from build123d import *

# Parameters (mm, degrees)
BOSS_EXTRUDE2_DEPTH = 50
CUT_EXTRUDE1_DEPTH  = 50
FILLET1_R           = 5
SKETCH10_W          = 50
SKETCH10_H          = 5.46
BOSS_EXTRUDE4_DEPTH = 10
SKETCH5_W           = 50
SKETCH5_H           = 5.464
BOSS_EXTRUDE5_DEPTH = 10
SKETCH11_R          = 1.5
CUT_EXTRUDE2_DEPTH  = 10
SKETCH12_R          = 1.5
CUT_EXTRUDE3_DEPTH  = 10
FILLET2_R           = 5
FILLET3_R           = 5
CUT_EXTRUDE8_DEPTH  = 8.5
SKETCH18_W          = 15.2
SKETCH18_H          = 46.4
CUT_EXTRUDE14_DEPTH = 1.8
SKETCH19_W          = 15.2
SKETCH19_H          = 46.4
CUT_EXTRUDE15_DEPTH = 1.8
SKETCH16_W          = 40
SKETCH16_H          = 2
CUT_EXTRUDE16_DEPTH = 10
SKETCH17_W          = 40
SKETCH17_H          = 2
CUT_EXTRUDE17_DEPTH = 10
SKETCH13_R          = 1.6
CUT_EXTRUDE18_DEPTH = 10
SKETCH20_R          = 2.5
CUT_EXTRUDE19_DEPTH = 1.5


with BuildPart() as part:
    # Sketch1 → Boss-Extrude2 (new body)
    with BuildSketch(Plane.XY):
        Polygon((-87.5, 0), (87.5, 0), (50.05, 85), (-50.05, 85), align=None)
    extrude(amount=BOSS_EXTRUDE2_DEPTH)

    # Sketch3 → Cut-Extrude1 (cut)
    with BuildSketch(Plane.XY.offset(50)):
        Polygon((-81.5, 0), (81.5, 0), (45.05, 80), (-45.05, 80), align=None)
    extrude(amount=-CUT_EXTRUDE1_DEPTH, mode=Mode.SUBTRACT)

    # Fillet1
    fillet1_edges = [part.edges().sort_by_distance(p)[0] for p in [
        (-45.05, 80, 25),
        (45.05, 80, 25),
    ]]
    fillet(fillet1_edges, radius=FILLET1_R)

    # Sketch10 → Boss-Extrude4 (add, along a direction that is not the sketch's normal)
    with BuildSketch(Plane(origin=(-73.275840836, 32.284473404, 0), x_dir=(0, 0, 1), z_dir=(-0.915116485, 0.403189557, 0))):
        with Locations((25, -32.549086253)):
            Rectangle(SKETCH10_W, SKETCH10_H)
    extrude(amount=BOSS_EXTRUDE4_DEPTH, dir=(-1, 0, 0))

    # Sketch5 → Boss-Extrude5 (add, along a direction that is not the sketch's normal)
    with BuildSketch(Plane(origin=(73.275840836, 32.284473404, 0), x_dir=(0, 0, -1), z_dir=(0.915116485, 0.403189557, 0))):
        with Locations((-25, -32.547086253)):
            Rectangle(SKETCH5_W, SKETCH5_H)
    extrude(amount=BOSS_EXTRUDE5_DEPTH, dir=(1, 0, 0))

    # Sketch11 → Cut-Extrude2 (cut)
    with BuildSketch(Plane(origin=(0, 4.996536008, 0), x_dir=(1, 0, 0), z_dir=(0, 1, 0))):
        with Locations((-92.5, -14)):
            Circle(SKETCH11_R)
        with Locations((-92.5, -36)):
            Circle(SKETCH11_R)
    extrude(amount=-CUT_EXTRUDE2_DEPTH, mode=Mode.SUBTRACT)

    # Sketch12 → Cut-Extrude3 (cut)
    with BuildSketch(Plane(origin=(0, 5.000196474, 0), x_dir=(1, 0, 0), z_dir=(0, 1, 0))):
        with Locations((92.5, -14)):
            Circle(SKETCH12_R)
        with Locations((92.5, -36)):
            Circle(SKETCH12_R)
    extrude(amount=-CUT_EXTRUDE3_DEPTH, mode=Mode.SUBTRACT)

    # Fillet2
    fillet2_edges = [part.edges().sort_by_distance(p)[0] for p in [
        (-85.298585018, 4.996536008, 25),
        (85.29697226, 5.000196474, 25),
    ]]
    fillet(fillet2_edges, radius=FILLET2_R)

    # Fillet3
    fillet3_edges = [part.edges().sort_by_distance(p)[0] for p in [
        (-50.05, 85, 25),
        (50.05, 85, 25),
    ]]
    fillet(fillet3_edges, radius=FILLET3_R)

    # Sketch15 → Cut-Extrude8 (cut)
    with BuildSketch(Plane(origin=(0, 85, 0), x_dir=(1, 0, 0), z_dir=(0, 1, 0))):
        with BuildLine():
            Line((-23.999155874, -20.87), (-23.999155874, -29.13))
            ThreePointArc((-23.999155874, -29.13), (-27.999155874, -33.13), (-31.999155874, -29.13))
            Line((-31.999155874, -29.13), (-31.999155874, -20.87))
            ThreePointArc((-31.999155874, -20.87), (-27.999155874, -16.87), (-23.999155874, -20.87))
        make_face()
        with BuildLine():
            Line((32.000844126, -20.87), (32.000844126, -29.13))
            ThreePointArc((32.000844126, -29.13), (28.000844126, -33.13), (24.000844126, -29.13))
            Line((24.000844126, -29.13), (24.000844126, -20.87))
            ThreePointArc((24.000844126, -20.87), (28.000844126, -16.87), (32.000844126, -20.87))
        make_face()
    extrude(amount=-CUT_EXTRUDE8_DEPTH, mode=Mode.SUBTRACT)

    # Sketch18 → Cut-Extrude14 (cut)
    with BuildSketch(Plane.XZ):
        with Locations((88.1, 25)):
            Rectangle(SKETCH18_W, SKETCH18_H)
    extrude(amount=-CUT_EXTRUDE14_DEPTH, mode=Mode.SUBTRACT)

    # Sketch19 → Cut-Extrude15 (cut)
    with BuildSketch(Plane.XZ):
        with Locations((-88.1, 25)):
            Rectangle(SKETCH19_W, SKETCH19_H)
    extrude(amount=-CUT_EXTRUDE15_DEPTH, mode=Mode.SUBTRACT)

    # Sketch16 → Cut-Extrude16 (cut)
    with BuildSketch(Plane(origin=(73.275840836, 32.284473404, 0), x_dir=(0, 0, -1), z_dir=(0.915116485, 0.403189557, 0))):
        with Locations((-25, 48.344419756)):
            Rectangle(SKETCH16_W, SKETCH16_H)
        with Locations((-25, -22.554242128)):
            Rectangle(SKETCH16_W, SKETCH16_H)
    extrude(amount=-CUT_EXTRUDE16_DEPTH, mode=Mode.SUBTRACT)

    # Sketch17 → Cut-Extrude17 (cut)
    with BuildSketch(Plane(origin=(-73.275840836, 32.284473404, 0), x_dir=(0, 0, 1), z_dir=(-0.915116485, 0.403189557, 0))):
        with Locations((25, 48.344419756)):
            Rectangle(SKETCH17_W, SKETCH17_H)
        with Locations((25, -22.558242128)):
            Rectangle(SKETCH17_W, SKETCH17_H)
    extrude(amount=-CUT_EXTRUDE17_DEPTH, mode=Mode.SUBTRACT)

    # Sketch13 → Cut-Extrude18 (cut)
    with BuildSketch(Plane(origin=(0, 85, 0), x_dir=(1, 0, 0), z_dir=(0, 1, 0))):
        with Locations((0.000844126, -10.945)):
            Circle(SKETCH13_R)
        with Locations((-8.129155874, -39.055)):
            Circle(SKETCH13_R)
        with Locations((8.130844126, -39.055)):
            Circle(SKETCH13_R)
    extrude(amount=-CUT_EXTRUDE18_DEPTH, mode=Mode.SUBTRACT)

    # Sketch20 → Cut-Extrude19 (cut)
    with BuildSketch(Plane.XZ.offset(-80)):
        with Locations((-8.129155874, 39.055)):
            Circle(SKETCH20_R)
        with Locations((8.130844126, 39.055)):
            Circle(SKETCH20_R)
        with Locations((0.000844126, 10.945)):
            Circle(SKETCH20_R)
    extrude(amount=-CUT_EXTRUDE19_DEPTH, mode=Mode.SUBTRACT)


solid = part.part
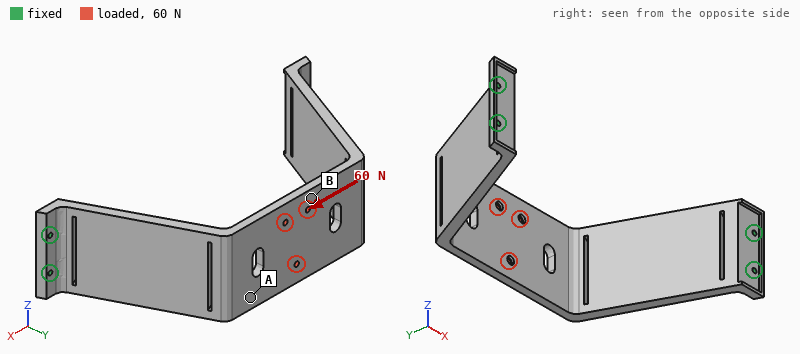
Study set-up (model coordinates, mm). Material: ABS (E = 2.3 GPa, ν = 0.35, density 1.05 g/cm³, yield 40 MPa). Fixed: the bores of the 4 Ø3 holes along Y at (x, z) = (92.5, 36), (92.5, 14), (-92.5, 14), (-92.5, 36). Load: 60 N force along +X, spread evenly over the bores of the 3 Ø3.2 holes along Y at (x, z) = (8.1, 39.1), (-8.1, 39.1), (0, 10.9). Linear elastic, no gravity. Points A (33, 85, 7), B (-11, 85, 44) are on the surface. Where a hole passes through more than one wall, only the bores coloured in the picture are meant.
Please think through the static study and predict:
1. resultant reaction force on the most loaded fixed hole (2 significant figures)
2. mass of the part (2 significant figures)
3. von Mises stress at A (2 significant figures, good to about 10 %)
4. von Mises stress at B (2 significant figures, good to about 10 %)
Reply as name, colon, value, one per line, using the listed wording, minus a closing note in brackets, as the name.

resultant reaction force on the most loaded fixed hole: 22 N
mass of the part: 82 g
von Mises stress at A: 4.2 MPa
von Mises stress at B: 1.6 MPa
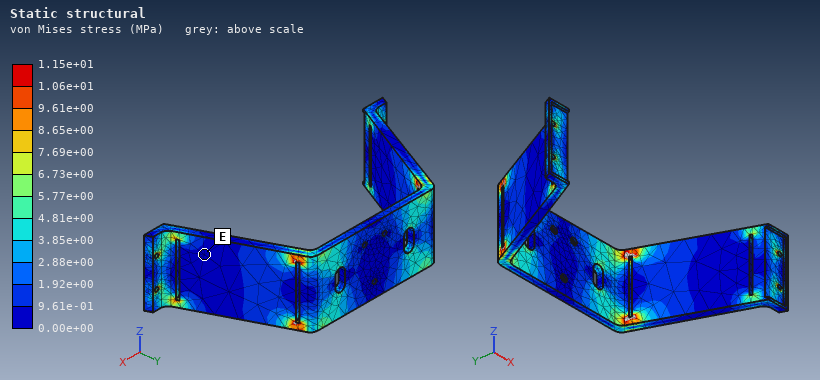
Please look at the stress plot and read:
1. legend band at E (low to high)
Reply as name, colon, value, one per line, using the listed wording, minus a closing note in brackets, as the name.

legend band at E: 0.00e+00 to 9.61e-01 MPa
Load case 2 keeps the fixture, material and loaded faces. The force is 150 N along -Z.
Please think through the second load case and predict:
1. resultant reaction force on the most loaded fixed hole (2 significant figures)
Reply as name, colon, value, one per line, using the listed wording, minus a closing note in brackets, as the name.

resultant reaction force on the most loaded fixed hole: 280 N
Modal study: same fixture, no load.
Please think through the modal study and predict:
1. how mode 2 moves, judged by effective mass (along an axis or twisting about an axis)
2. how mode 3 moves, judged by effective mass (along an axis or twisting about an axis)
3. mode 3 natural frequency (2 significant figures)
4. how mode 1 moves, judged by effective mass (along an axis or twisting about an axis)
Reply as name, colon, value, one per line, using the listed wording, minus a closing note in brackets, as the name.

how mode 2 moves, judged by effective mass: along Z
how mode 3 moves, judged by effective mass: twisting about Y
mode 3 natural frequency: 290 Hz
how mode 1 moves, judged by effective mass: along X
